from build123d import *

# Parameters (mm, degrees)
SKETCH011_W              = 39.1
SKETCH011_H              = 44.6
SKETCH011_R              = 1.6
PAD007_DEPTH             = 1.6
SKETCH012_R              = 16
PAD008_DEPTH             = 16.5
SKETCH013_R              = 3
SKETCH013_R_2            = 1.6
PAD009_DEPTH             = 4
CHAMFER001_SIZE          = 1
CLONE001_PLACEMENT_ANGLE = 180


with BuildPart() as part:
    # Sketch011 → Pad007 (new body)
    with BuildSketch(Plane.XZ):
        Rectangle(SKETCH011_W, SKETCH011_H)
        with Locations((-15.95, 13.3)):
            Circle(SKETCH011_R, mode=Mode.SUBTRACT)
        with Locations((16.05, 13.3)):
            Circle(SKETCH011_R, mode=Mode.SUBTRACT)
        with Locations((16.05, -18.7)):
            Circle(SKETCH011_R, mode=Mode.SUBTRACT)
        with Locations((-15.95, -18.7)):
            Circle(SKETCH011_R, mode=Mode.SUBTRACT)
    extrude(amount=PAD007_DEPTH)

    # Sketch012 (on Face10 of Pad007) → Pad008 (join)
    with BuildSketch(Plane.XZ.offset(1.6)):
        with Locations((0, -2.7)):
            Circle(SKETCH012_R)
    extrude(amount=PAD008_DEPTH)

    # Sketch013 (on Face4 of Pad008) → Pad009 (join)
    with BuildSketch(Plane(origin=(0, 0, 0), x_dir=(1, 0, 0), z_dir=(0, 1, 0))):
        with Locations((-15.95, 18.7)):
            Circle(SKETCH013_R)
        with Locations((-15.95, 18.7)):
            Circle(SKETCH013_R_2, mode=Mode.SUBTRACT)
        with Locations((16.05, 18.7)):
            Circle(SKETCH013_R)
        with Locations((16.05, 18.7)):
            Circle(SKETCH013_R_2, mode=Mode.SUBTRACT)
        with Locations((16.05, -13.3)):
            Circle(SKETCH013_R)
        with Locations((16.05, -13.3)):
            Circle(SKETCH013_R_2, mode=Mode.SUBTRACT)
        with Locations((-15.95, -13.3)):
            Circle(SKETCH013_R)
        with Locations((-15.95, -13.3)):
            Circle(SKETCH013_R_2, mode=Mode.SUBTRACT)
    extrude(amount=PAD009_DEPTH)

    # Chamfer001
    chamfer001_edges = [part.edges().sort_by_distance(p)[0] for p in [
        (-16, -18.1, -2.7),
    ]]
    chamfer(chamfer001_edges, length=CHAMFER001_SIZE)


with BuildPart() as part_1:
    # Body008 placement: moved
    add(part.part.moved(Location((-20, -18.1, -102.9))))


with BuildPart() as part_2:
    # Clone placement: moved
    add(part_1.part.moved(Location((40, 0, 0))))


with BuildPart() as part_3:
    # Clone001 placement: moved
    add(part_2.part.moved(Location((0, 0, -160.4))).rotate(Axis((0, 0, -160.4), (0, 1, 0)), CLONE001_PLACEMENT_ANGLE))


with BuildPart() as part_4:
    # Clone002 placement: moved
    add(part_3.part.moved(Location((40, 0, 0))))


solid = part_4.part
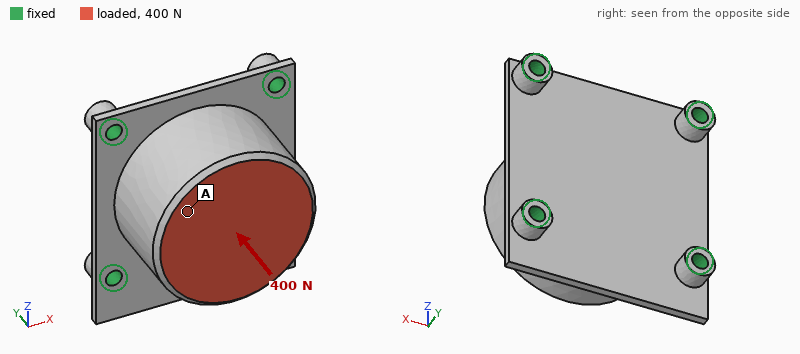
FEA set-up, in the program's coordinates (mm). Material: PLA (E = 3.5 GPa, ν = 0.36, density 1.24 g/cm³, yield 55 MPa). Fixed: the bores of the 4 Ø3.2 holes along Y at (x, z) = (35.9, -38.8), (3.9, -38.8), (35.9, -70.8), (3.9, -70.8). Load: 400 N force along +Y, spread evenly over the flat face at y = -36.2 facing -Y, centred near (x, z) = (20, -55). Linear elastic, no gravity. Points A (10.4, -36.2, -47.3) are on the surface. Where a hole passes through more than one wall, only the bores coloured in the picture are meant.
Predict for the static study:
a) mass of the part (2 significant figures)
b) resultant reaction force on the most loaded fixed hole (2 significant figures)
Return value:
20 g
120 N
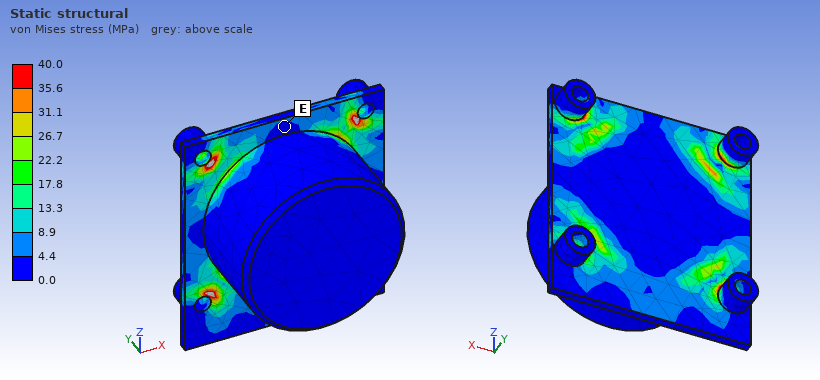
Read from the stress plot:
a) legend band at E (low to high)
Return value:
0.0 to 4.4 MPa
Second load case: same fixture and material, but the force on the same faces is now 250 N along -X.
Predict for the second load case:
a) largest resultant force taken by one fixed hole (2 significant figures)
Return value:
110 N
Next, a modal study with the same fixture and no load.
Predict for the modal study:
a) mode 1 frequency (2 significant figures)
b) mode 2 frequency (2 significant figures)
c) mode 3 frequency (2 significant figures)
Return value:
1900 Hz
2000 Hz
2000 Hz
